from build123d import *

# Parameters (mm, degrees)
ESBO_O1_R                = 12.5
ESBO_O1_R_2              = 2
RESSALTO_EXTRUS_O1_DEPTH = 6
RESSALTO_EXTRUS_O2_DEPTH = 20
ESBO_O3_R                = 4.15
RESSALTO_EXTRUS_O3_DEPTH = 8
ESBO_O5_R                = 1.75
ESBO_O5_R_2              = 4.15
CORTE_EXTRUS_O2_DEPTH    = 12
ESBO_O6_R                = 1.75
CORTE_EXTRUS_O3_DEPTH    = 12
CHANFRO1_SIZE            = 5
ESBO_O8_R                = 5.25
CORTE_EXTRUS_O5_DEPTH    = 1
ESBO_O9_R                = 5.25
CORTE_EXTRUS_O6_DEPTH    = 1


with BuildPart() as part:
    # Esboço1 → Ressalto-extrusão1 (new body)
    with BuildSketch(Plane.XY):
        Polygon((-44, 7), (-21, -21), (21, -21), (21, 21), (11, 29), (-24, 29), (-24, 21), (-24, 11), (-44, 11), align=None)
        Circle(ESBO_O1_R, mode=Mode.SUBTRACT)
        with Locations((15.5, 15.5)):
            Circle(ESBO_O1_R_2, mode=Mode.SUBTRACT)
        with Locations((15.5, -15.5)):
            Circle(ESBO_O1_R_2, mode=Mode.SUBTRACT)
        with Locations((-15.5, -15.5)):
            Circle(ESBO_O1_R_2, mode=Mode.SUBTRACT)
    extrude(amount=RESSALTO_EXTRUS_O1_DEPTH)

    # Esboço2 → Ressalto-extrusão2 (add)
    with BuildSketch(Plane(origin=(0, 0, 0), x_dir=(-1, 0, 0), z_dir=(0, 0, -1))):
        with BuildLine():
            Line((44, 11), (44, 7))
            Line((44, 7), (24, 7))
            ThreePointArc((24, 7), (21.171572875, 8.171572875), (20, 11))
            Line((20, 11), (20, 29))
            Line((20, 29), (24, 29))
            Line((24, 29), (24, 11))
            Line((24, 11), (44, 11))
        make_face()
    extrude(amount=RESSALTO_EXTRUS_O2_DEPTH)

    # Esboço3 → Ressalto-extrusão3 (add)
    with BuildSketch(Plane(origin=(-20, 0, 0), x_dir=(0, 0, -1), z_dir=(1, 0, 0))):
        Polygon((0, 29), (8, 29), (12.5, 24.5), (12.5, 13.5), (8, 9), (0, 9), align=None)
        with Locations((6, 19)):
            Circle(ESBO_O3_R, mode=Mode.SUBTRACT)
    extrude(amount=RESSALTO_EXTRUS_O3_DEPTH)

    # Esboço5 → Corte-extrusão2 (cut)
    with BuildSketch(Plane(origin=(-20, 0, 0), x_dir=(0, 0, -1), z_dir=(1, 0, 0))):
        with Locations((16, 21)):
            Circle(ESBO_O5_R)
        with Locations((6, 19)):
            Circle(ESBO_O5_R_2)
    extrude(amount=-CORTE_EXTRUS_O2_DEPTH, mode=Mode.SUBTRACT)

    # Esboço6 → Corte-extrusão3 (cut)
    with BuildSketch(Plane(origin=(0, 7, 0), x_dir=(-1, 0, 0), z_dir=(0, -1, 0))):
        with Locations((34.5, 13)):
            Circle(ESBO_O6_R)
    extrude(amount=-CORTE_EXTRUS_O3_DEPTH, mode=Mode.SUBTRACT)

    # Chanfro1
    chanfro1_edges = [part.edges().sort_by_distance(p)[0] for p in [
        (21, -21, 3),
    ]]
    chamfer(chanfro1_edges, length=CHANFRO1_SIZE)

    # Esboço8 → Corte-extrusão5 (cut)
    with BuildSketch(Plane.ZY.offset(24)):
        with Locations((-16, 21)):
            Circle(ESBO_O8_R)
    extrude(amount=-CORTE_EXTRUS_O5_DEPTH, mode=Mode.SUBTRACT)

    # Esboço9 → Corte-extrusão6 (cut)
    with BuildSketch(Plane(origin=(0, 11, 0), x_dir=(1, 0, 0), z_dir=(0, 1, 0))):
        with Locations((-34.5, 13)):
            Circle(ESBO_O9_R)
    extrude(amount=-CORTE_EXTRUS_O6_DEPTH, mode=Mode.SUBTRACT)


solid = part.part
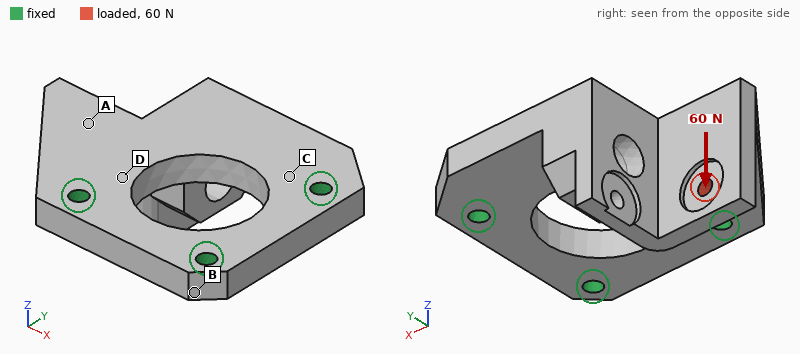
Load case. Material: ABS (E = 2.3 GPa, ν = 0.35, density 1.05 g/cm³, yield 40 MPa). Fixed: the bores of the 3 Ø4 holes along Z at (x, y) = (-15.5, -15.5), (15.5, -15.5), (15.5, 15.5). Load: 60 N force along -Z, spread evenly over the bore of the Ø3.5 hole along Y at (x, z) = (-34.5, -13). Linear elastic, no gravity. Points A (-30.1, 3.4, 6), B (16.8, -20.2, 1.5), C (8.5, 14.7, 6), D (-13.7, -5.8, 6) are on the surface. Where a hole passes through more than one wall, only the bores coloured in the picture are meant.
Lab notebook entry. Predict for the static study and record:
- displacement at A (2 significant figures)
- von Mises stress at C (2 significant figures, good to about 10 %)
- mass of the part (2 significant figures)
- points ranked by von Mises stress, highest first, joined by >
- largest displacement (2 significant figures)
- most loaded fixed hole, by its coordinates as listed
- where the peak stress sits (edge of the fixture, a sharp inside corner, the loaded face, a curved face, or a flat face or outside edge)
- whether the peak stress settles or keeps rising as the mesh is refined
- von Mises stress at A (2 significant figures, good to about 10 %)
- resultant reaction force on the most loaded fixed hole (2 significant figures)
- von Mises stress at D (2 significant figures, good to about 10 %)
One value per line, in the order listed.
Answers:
0.36 mm
4.7 MPa
17 g
D > C > A > B
0.86 mm
(-15.5, -15.5)
edge of the fixture
keeps rising
2.5 MPa
61 N
7.7 MPa
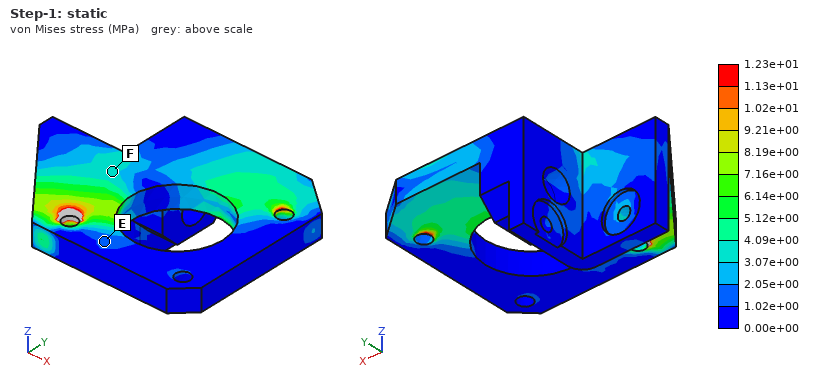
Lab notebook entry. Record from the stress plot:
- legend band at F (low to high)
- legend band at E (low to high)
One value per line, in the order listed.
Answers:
3.07e+00 to 4.09e+00 MPa
1.02e+00 to 2.05e+00 MPa
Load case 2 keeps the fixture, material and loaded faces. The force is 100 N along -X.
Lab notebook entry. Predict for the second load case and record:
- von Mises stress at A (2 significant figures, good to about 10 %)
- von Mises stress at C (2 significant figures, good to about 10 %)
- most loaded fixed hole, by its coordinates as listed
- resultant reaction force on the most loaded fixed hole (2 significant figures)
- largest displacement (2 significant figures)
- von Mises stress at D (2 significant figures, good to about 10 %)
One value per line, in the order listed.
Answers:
3.5 MPa
2.9 MPa
(15.5, 15.5)
77 N
0.89 mm
6.6 MPa
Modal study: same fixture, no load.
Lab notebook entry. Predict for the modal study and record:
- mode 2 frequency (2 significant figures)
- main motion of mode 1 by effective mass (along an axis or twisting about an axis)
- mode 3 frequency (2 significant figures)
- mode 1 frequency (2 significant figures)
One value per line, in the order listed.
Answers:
1600 Hz
along Z
2400 Hz
670 Hz
